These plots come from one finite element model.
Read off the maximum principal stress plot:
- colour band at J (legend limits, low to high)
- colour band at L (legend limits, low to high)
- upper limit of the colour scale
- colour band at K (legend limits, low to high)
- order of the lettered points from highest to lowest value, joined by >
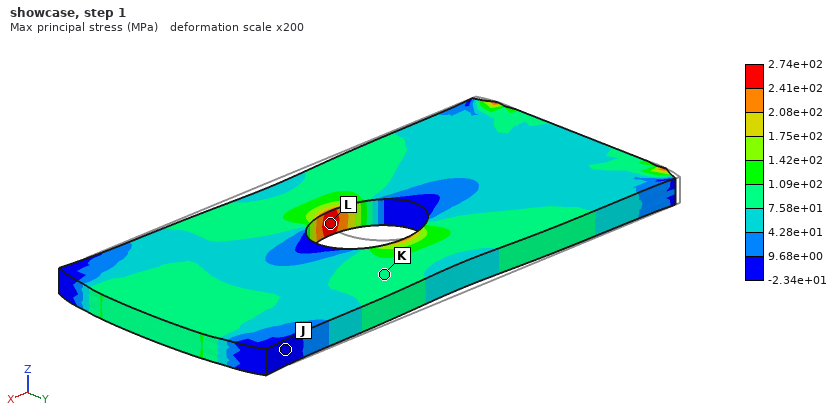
-2.34e+01 to 9.68e+00 MPa
2.41e+02 to 2.74e+02 MPa
2.74e+02 MPa
7.58e+01 to 1.09e+02 MPa
L > K > J
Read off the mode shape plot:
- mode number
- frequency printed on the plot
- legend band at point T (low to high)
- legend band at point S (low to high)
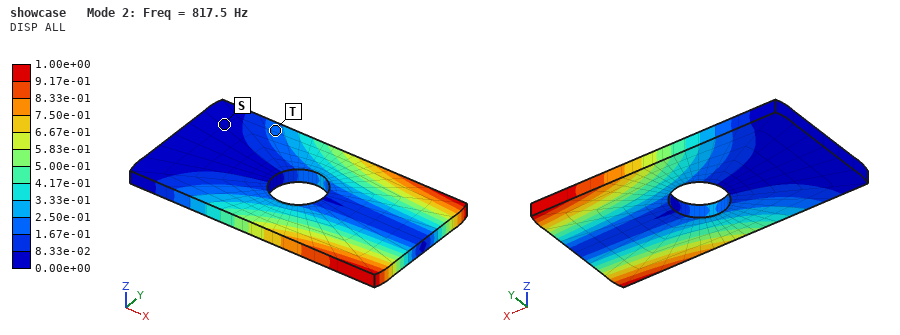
2
817.5 Hz
1.67e-01 to 2.50e-01
0.00e+00 to 8.33e-02
